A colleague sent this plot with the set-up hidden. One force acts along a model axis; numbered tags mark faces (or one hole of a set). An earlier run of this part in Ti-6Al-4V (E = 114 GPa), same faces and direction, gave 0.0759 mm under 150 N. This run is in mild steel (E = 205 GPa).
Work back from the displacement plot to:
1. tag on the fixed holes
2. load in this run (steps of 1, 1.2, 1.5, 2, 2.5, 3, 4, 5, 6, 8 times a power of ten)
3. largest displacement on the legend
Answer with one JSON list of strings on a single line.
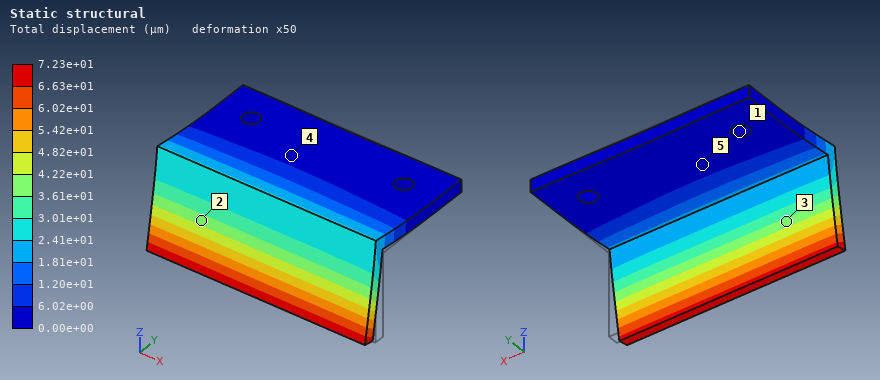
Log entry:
["1", "250 N", "7.23e+01 µm"]
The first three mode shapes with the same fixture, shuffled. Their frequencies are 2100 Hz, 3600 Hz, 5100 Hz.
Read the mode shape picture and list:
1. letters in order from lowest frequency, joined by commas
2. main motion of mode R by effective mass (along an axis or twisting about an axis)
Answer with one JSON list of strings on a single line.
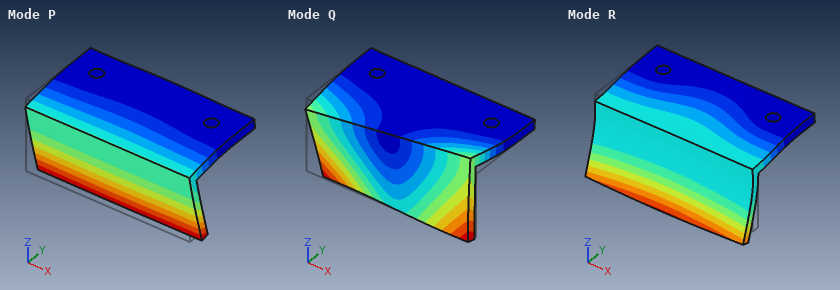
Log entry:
["P, Q, R", "along Z"]
